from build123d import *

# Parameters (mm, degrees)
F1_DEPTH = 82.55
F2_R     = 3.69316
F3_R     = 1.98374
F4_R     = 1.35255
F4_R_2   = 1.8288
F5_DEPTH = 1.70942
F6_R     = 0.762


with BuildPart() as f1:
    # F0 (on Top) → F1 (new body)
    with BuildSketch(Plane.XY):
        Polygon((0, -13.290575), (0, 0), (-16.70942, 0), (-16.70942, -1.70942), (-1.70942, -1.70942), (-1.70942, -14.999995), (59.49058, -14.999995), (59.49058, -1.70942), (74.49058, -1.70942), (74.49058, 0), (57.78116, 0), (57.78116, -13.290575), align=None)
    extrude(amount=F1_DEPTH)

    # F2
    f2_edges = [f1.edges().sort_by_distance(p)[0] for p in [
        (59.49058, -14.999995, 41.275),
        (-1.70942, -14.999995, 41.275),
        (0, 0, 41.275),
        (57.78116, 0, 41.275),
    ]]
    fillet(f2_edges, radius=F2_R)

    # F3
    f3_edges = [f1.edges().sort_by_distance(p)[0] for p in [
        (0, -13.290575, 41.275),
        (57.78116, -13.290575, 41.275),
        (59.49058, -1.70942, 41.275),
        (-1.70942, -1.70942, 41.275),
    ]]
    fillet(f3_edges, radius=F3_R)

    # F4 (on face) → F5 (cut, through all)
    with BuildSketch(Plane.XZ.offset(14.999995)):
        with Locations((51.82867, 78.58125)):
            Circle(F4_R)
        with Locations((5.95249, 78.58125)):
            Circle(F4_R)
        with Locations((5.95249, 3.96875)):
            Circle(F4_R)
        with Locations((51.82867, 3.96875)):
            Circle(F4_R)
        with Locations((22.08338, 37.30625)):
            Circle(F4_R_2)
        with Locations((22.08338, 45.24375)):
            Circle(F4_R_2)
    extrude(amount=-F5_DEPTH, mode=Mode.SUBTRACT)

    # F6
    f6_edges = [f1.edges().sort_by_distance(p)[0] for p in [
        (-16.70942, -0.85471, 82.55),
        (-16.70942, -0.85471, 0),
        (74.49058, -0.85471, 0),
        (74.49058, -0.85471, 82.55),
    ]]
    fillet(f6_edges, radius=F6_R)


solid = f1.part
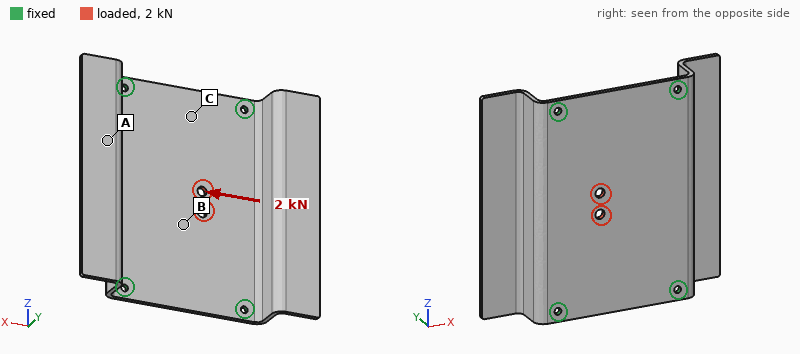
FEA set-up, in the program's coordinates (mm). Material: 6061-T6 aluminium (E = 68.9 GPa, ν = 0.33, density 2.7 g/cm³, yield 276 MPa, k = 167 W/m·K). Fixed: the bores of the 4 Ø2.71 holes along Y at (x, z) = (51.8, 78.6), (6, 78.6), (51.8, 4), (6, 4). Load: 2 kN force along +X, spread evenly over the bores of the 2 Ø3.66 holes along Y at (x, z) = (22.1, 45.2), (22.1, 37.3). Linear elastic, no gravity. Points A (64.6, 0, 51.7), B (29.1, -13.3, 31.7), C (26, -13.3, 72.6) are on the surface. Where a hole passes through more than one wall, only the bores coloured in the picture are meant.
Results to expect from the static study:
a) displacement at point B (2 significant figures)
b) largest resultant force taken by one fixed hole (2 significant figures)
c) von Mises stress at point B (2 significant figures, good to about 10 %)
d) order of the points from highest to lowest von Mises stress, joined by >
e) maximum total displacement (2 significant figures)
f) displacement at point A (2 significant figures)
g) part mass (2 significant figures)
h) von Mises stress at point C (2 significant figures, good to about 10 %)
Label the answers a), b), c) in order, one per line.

a) 18 µm
b) 600 N
c) 29 MPa
d) B > C > A
e) 26 µm
f) 19 µm
g) 43 g
h) 17 MPa
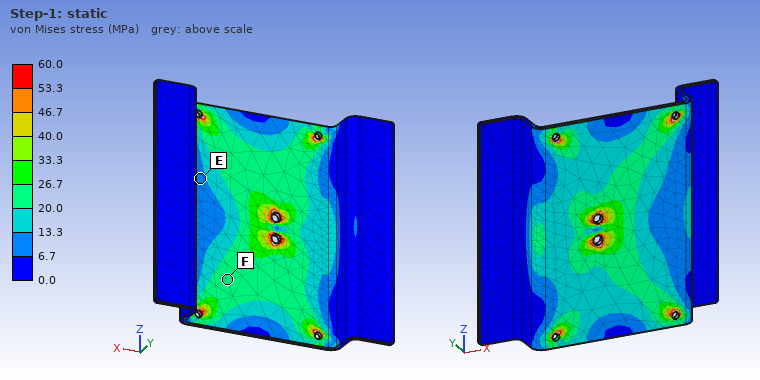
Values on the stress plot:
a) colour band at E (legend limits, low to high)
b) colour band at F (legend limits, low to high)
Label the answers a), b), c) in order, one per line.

a) 6.7 to 13.3 MPa
b) 20.0 to 26.7 MPa
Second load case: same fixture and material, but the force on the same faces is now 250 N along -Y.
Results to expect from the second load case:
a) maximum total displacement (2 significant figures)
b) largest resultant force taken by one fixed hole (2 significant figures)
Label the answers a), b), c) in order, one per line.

a) 0.28 mm
b) 120 N
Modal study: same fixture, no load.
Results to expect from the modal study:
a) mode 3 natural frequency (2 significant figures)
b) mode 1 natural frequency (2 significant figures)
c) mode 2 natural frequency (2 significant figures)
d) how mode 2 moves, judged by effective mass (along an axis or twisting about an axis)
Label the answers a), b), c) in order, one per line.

a) 2100 Hz
b) 1300 Hz
c) 1400 Hz
d) along X
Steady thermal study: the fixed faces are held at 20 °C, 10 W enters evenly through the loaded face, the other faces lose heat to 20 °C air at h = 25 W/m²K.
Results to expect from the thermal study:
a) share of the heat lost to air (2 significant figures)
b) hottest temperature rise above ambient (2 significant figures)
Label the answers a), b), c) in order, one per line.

a) 22 %
b) 18 K
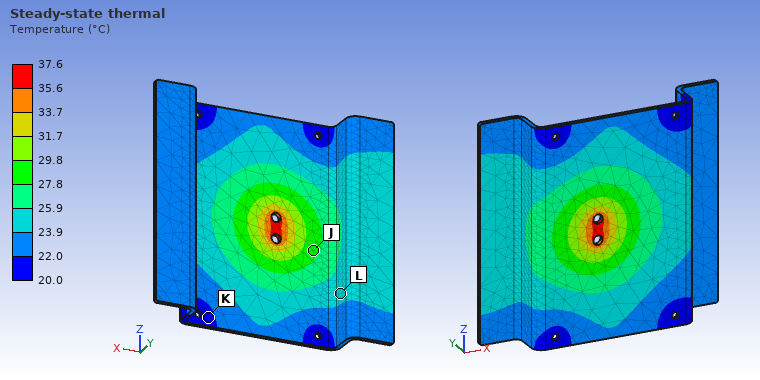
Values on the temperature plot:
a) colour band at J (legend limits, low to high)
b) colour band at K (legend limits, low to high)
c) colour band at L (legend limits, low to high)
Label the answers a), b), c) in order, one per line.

a) 27.8 to 29.8 °C
b) 20.0 to 22.0 °C
c) 23.9 to 25.9 °C
